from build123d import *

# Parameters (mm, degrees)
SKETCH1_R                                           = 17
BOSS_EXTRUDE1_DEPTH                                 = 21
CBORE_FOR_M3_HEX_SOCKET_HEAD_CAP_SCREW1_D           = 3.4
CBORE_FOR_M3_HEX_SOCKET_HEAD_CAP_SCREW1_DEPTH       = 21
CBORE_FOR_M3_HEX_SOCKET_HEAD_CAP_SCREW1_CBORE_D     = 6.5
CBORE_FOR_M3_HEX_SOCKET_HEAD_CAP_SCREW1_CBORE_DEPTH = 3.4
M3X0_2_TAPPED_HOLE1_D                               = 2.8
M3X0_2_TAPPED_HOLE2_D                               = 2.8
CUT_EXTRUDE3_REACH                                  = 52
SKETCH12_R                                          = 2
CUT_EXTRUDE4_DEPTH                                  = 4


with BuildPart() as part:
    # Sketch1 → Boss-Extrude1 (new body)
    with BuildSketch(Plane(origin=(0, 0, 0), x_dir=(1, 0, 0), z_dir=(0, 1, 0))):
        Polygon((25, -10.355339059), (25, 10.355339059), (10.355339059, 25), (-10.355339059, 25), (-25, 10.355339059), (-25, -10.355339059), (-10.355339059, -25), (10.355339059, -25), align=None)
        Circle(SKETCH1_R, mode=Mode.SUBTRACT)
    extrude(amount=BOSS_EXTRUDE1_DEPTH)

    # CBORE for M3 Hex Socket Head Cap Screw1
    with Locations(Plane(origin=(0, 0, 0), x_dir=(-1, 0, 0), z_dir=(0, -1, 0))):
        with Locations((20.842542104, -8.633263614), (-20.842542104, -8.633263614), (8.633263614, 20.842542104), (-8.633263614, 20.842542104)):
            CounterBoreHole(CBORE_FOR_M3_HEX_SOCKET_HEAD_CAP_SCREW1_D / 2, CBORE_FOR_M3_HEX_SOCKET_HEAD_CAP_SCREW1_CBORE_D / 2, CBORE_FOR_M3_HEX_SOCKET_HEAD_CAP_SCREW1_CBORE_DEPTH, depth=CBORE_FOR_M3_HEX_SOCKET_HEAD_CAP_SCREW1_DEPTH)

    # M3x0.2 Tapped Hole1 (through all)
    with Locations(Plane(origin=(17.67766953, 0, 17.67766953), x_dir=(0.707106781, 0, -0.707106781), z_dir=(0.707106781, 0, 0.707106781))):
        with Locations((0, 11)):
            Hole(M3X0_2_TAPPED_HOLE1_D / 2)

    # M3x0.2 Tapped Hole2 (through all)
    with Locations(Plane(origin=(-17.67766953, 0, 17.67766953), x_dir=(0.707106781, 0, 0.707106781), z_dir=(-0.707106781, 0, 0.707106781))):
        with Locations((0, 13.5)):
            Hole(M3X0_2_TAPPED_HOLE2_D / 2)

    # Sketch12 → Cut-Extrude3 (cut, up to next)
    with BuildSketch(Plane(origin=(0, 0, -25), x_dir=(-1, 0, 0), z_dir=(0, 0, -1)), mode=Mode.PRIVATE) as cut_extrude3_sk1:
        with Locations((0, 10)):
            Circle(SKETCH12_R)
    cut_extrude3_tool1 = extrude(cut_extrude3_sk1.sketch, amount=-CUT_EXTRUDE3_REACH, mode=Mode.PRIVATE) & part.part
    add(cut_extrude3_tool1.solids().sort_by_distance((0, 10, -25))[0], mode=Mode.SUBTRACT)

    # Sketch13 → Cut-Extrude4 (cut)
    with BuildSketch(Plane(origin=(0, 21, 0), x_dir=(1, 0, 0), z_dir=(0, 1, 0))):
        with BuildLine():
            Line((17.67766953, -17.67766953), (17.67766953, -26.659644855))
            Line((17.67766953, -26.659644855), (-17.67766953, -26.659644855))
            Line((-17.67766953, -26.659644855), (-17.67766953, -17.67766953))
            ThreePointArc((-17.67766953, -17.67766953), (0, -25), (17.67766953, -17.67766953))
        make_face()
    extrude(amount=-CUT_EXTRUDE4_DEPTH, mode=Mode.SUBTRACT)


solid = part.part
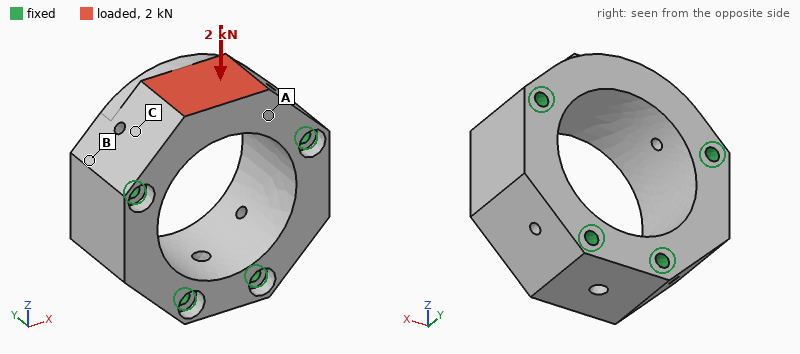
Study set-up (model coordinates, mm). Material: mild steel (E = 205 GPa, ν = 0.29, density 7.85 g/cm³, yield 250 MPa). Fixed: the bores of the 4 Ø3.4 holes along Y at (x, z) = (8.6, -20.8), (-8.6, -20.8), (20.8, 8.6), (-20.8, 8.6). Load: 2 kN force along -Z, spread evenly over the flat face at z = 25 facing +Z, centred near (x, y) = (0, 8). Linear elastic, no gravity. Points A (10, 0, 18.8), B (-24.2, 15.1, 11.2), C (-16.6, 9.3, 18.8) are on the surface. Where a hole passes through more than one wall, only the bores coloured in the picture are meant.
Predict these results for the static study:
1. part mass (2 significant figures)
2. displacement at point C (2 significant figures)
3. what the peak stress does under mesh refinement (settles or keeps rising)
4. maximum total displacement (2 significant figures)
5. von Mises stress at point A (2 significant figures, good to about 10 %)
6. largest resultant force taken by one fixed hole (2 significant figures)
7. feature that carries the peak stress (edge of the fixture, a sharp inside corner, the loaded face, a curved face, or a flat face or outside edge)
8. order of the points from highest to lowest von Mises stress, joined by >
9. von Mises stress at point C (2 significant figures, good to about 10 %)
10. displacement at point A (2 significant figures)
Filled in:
180 g
0.54 µm
keeps rising
2.9 µm
13 MPa
1.3 kN
edge of the fixture
A > C > B
6.1 MPa
1.7 µm
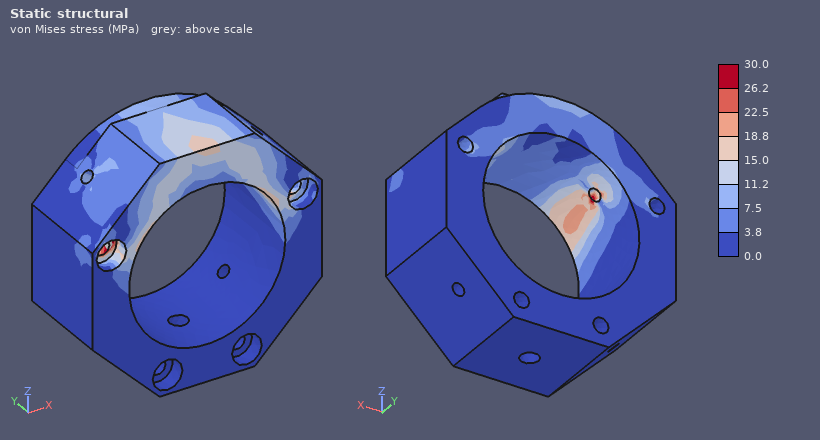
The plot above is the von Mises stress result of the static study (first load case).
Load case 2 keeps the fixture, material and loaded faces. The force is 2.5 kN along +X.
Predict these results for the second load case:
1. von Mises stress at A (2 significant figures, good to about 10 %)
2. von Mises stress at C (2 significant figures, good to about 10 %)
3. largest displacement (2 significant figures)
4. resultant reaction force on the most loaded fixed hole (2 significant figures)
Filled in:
6.7 MPa
10.0 MPa
1.8 µm
1.5 kN
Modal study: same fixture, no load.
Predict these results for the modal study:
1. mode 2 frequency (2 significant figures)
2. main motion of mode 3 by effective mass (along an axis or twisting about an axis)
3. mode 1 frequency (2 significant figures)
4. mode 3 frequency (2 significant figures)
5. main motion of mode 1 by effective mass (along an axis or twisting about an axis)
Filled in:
27 kHz
along Z
19 kHz
30 kHz
along Y
